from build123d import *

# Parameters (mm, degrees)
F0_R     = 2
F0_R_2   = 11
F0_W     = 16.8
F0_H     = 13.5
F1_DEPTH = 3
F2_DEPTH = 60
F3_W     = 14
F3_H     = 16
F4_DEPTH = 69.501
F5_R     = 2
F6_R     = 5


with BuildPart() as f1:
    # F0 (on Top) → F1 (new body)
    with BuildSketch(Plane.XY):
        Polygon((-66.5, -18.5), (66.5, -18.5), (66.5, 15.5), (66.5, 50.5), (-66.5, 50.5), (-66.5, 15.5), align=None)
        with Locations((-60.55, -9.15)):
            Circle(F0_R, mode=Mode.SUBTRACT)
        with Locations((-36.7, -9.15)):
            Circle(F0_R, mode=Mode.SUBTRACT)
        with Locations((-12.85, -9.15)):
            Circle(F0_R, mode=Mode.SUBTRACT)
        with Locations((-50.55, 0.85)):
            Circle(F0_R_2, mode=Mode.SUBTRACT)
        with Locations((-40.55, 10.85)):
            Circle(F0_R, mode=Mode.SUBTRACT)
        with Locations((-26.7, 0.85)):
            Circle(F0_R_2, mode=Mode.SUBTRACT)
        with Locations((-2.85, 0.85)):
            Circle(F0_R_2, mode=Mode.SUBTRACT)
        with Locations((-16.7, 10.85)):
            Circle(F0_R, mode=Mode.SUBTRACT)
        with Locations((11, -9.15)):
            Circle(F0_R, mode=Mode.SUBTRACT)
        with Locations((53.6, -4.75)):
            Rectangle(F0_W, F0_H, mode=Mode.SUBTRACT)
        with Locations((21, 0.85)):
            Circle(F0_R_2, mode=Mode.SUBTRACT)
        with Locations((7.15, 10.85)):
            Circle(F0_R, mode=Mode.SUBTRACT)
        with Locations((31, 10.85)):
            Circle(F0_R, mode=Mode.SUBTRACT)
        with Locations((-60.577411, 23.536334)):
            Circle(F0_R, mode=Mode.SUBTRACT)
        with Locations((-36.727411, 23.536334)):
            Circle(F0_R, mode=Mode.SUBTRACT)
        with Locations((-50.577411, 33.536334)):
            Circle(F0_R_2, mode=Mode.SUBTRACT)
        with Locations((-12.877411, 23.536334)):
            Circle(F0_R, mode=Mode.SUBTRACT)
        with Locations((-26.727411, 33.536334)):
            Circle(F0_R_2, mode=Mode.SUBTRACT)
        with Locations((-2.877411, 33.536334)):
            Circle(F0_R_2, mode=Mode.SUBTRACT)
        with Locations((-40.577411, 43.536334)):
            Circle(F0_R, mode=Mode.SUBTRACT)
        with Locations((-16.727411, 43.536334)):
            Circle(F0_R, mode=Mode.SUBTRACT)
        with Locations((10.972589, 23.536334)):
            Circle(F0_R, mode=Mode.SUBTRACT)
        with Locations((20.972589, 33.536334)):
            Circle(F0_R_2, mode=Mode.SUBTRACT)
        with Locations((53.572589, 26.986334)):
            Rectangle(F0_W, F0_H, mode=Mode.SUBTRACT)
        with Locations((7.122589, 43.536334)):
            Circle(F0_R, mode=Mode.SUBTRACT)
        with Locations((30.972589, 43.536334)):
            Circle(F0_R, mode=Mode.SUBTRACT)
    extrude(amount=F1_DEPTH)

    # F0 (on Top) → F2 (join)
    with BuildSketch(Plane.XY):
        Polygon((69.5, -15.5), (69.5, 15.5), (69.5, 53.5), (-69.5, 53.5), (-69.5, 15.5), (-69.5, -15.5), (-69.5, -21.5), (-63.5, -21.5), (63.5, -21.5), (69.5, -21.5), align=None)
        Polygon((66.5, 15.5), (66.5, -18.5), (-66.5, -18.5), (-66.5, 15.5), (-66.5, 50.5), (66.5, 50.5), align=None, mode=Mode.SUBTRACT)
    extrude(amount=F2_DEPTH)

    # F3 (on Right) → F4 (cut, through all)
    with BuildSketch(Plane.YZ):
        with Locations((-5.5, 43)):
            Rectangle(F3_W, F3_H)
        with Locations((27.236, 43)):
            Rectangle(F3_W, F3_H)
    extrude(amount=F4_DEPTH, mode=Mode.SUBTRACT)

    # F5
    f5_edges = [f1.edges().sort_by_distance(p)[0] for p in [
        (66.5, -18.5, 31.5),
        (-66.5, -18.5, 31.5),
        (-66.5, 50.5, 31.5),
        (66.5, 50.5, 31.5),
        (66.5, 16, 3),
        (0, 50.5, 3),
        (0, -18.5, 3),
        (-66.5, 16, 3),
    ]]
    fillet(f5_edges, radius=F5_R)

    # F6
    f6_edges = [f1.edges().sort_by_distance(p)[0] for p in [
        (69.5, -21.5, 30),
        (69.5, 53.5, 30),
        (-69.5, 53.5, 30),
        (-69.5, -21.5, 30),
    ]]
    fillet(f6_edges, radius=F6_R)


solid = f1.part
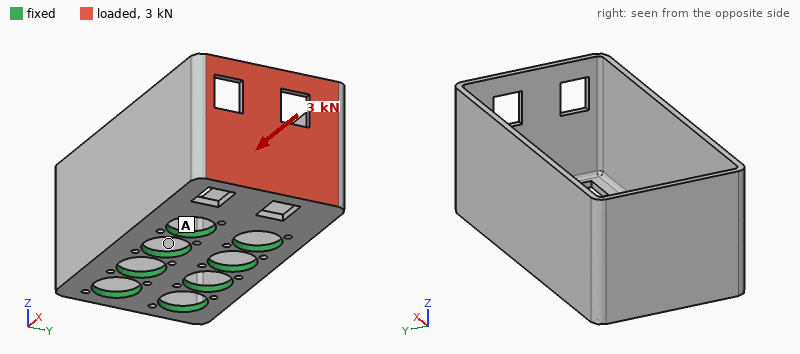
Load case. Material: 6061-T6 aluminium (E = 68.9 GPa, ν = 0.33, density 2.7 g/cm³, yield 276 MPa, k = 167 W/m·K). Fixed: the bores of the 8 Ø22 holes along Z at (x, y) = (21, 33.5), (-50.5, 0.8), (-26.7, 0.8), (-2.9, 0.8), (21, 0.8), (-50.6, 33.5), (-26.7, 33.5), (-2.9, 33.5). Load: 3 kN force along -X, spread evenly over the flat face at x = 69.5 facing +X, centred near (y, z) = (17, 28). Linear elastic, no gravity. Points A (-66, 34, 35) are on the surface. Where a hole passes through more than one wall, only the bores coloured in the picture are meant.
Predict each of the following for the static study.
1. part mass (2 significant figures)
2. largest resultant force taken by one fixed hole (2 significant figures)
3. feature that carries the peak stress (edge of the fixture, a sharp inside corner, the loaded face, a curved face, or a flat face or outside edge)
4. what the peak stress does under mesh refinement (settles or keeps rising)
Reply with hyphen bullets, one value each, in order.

- 240 g
- 940 N
- a sharp inside corner
- keeps rising
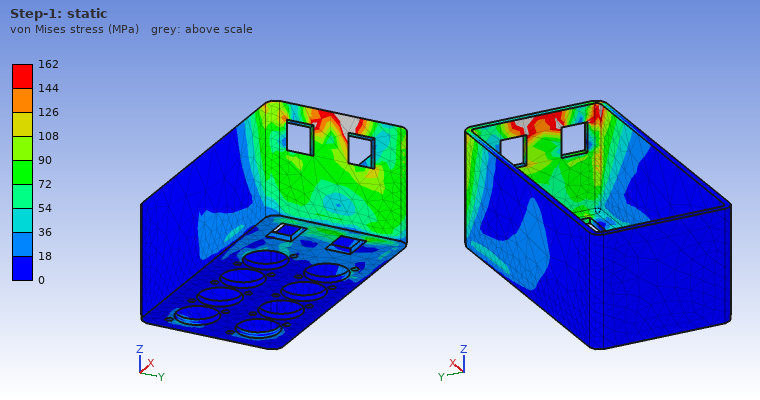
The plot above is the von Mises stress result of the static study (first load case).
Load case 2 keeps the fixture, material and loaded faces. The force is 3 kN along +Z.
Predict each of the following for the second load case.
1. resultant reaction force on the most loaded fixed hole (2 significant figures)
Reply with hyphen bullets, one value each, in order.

- 2.1 kN
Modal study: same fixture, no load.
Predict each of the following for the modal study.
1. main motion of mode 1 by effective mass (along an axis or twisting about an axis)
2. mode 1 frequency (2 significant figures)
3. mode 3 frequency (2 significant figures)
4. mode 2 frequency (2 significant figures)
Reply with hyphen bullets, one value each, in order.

- along Y
- 1000 Hz
- 1700 Hz
- 1100 Hz
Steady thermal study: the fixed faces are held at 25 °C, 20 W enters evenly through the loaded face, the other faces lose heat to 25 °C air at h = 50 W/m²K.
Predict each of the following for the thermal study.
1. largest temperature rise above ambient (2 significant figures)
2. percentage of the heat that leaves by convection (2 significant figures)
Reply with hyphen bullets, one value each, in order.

- 15 K
- 41 %
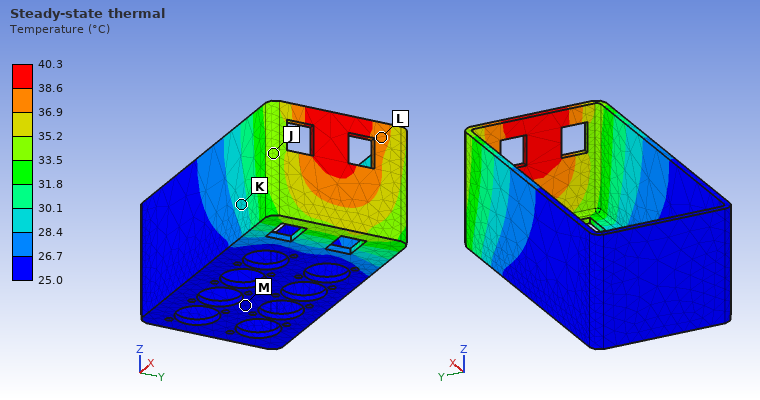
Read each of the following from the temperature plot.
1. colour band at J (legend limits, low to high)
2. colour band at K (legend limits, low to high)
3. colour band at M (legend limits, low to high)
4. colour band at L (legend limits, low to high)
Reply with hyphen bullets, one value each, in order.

- 33.5 to 35.2 °C
- 28.4 to 30.1 °C
- 25.0 to 26.7 °C
- 36.9 to 38.6 °C
